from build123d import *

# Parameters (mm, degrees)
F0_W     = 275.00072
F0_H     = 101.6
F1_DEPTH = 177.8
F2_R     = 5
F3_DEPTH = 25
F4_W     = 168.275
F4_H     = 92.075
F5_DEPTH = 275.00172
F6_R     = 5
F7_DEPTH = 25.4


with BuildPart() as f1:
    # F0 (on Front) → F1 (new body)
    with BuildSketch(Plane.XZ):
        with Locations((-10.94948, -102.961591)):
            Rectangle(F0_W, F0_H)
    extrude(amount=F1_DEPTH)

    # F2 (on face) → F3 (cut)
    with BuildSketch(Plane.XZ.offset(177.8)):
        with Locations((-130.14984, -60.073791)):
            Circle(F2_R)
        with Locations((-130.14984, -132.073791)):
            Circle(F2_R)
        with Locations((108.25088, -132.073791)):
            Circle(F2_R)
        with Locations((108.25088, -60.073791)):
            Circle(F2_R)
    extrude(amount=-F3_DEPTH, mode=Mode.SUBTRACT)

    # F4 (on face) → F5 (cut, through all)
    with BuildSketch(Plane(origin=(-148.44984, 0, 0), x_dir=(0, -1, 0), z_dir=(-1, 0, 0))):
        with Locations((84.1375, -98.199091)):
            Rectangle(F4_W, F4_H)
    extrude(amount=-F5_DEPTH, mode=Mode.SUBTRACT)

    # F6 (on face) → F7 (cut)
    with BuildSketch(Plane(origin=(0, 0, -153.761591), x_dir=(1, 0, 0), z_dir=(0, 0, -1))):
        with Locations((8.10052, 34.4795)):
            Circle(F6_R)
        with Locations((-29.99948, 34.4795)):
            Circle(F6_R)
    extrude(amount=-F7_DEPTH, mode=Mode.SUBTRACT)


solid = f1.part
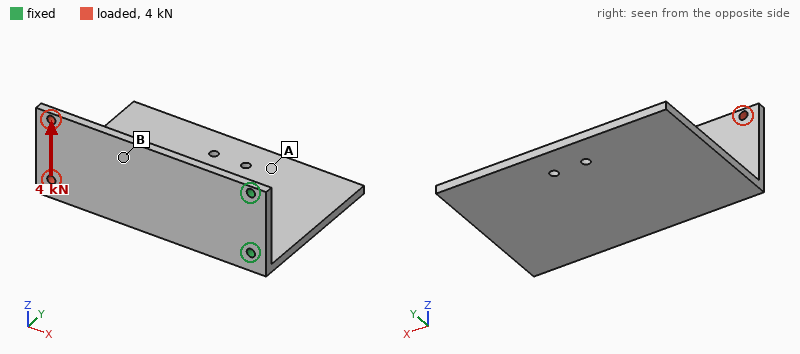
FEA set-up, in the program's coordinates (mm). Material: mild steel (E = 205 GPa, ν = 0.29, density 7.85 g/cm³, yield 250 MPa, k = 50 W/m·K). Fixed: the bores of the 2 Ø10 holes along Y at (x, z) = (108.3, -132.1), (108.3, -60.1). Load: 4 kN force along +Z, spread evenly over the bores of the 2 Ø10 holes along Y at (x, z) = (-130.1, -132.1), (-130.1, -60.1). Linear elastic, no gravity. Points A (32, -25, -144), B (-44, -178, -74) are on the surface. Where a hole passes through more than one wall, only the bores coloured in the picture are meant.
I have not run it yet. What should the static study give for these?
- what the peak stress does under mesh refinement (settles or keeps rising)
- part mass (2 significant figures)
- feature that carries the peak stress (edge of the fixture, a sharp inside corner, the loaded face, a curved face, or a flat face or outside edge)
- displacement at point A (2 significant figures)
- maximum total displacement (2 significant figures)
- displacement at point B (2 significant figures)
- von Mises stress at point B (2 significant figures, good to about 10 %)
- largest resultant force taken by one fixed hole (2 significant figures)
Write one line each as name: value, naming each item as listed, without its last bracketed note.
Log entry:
what the peak stress does under mesh refinement: keeps rising
part mass: 5.5 kg
feature that carries the peak stress: edge of the fixture
displacement at point A: 0.025 mm
maximum total displacement: 0.12 mm
displacement at point B: 0.060 mm
von Mises stress at point B: 11 MPa
largest resultant force taken by one fixed hole: 13 kN
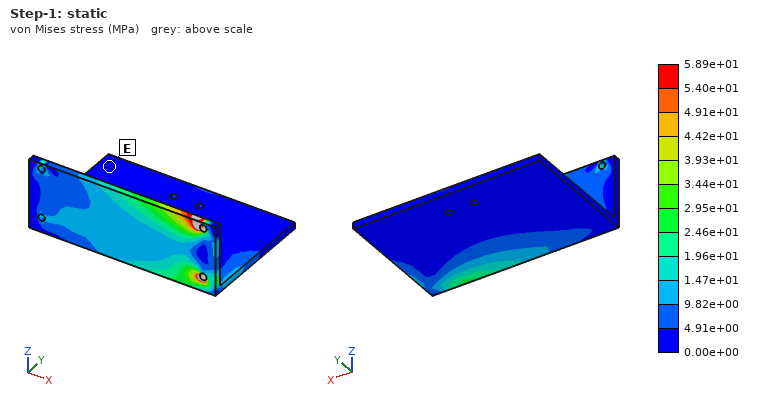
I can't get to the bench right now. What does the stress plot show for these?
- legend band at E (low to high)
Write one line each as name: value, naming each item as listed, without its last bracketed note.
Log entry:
legend band at E: 0.00e+00 to 4.91e+00 MPa
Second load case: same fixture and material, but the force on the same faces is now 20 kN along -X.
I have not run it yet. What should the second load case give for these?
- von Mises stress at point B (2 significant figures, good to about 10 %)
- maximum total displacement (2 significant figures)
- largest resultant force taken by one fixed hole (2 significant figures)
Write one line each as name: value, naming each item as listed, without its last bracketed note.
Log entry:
von Mises stress at point B: 27 MPa
maximum total displacement: 64 µm
largest resultant force taken by one fixed hole: 10 kN
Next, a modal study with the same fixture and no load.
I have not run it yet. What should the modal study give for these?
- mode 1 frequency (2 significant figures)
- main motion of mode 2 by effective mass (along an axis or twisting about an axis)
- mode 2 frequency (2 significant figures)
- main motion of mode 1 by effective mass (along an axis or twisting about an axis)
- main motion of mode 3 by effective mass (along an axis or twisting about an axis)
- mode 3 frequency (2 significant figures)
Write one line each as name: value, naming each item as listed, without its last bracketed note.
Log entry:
mode 1 frequency: 120 Hz
main motion of mode 2 by effective mass: along Z
mode 2 frequency: 150 Hz
main motion of mode 1 by effective mass: along Y
main motion of mode 3 by effective mass: twisting about Y
mode 3 frequency: 390 Hz
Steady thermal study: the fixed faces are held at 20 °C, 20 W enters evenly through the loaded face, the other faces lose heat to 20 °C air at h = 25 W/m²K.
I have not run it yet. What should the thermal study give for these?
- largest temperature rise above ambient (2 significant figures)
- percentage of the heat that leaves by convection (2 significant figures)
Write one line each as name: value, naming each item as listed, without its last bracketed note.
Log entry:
largest temperature rise above ambient: 34 K
percentage of the heat that leaves by convection: 92 %
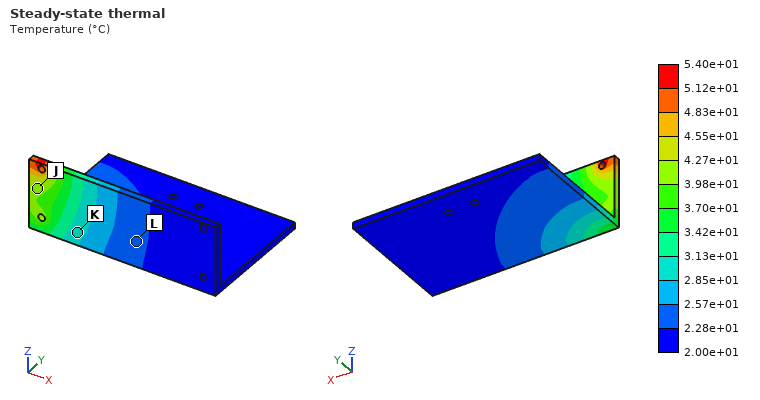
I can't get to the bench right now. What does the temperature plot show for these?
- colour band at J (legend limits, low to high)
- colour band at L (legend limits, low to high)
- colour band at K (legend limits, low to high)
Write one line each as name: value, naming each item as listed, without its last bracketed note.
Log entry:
colour band at J: 3.98e+01 to 4.27e+01 °C
colour band at L: 2.28e+01 to 2.57e+01 °C
colour band at K: 2.85e+01 to 3.13e+01 °C
